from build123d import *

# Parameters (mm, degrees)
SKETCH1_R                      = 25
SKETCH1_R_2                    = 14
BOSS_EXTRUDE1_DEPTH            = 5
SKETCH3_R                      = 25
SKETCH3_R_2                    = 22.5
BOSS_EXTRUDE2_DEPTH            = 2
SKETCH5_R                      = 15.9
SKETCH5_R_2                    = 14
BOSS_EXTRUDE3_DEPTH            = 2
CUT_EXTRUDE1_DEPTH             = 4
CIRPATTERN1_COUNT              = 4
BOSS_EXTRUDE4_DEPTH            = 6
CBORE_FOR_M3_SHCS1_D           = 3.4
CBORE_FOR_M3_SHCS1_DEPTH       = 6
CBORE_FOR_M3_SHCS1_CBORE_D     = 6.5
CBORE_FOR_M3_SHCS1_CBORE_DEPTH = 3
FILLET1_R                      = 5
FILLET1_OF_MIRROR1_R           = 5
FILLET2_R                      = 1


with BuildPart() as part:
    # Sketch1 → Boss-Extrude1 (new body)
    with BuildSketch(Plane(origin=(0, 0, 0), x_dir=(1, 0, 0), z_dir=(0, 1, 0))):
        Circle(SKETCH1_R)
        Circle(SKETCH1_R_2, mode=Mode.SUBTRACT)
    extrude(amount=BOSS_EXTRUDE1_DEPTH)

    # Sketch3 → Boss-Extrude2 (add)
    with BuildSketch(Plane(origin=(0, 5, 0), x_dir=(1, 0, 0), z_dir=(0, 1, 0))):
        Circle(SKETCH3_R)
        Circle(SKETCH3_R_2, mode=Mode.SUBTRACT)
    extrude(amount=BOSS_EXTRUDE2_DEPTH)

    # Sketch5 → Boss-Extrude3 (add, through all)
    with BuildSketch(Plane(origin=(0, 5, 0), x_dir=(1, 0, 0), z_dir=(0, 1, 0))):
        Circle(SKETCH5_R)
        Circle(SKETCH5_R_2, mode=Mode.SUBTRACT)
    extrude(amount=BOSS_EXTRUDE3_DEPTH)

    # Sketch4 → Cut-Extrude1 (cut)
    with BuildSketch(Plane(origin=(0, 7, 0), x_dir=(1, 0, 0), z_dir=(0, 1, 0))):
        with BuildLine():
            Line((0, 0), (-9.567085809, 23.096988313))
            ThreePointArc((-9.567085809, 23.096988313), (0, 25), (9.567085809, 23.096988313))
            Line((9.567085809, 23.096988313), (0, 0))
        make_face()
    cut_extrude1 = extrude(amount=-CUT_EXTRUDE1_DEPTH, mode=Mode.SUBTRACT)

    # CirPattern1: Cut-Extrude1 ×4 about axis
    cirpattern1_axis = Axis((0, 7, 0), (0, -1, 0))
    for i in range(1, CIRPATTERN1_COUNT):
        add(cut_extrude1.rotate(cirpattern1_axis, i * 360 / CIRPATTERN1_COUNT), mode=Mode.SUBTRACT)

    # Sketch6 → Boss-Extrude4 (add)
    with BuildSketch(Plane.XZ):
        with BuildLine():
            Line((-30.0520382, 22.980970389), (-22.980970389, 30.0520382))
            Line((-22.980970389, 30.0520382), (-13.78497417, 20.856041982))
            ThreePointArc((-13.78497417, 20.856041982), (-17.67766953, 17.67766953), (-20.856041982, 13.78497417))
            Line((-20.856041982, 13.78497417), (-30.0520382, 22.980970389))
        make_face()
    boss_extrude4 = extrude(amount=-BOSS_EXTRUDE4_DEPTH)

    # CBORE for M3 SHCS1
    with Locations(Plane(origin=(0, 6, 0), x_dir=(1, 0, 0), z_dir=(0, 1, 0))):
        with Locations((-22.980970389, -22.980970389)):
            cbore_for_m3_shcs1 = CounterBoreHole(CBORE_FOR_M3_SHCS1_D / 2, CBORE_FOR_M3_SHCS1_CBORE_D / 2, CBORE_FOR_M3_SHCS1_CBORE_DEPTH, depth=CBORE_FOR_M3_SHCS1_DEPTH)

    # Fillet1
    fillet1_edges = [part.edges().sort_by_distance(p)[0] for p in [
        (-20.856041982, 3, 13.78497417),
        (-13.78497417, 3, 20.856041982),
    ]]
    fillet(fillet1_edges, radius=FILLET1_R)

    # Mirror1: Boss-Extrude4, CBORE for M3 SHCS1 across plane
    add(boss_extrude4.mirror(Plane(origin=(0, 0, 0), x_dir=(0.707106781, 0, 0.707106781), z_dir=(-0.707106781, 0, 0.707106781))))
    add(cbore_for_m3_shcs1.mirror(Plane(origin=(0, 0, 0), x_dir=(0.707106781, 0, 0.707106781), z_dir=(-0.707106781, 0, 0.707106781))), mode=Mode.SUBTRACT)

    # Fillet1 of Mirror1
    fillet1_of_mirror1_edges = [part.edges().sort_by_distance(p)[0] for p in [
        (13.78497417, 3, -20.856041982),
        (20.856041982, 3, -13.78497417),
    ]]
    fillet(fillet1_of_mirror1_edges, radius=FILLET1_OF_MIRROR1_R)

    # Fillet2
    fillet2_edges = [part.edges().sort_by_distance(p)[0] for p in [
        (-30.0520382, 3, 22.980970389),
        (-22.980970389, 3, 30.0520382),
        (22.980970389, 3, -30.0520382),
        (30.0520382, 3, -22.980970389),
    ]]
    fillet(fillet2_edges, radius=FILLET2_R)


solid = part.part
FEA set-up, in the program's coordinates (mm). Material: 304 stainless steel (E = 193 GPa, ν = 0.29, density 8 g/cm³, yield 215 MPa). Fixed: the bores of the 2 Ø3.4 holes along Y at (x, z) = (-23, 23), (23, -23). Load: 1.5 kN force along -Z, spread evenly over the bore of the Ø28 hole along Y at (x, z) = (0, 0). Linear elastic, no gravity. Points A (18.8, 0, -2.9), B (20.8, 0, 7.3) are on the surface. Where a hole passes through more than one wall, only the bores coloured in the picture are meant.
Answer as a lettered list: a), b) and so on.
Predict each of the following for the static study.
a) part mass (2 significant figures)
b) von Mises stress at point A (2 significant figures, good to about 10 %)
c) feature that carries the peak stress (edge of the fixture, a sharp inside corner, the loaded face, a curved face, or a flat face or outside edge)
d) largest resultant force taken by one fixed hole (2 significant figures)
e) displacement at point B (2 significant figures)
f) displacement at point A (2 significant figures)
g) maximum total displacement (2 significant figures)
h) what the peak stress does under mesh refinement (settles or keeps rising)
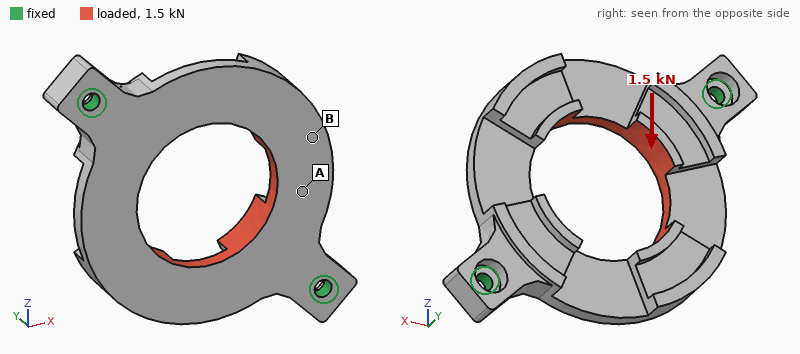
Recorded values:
a) 58 g
b) 22 MPa
c) edge of the fixture
d) 750 N
e) 6.6 µm
f) 3.8 µm
g) 14 µm
h) keeps rising
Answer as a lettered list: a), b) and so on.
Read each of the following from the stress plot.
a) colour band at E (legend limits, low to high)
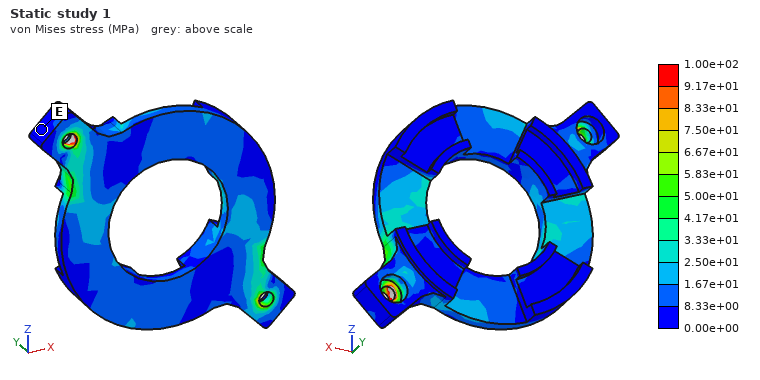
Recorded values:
a) 0.00e+00 to 8.33e+00 MPa
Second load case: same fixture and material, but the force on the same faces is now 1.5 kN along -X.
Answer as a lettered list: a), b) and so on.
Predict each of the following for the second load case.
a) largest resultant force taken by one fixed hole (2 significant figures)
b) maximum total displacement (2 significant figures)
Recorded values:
a) 750 N
b) 14 µm
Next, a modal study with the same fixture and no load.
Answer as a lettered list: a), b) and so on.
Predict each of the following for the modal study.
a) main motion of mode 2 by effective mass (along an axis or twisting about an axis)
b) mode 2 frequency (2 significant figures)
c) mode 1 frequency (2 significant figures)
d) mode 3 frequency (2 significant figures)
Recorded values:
a) along Y
b) 2900 Hz
c) 2600 Hz
d) 7100 Hz
